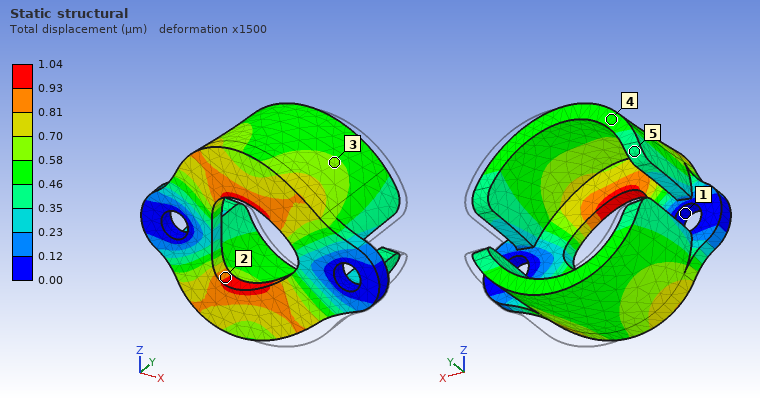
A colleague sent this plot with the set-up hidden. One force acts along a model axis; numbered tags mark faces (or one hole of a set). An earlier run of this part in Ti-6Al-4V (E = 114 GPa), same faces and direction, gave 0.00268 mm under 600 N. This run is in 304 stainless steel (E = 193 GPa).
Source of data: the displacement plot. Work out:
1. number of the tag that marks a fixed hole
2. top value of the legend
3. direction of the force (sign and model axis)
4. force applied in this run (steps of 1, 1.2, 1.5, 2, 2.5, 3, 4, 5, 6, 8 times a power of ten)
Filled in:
1
1.04 µm
-X
400 N
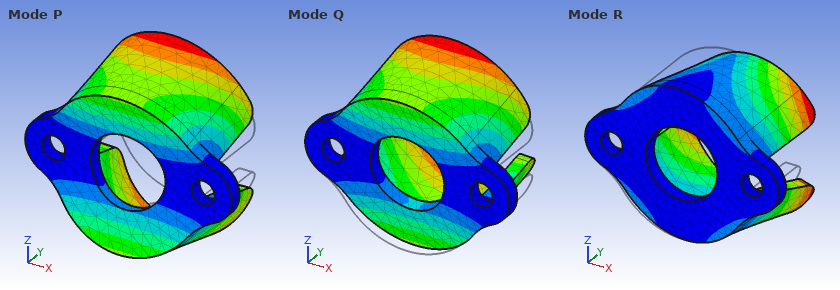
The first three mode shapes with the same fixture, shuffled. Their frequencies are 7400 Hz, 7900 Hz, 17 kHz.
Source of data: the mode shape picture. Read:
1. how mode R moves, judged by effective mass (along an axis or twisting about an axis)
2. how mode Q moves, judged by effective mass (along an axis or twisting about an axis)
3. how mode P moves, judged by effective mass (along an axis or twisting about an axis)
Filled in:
along X
along Z
along Y
